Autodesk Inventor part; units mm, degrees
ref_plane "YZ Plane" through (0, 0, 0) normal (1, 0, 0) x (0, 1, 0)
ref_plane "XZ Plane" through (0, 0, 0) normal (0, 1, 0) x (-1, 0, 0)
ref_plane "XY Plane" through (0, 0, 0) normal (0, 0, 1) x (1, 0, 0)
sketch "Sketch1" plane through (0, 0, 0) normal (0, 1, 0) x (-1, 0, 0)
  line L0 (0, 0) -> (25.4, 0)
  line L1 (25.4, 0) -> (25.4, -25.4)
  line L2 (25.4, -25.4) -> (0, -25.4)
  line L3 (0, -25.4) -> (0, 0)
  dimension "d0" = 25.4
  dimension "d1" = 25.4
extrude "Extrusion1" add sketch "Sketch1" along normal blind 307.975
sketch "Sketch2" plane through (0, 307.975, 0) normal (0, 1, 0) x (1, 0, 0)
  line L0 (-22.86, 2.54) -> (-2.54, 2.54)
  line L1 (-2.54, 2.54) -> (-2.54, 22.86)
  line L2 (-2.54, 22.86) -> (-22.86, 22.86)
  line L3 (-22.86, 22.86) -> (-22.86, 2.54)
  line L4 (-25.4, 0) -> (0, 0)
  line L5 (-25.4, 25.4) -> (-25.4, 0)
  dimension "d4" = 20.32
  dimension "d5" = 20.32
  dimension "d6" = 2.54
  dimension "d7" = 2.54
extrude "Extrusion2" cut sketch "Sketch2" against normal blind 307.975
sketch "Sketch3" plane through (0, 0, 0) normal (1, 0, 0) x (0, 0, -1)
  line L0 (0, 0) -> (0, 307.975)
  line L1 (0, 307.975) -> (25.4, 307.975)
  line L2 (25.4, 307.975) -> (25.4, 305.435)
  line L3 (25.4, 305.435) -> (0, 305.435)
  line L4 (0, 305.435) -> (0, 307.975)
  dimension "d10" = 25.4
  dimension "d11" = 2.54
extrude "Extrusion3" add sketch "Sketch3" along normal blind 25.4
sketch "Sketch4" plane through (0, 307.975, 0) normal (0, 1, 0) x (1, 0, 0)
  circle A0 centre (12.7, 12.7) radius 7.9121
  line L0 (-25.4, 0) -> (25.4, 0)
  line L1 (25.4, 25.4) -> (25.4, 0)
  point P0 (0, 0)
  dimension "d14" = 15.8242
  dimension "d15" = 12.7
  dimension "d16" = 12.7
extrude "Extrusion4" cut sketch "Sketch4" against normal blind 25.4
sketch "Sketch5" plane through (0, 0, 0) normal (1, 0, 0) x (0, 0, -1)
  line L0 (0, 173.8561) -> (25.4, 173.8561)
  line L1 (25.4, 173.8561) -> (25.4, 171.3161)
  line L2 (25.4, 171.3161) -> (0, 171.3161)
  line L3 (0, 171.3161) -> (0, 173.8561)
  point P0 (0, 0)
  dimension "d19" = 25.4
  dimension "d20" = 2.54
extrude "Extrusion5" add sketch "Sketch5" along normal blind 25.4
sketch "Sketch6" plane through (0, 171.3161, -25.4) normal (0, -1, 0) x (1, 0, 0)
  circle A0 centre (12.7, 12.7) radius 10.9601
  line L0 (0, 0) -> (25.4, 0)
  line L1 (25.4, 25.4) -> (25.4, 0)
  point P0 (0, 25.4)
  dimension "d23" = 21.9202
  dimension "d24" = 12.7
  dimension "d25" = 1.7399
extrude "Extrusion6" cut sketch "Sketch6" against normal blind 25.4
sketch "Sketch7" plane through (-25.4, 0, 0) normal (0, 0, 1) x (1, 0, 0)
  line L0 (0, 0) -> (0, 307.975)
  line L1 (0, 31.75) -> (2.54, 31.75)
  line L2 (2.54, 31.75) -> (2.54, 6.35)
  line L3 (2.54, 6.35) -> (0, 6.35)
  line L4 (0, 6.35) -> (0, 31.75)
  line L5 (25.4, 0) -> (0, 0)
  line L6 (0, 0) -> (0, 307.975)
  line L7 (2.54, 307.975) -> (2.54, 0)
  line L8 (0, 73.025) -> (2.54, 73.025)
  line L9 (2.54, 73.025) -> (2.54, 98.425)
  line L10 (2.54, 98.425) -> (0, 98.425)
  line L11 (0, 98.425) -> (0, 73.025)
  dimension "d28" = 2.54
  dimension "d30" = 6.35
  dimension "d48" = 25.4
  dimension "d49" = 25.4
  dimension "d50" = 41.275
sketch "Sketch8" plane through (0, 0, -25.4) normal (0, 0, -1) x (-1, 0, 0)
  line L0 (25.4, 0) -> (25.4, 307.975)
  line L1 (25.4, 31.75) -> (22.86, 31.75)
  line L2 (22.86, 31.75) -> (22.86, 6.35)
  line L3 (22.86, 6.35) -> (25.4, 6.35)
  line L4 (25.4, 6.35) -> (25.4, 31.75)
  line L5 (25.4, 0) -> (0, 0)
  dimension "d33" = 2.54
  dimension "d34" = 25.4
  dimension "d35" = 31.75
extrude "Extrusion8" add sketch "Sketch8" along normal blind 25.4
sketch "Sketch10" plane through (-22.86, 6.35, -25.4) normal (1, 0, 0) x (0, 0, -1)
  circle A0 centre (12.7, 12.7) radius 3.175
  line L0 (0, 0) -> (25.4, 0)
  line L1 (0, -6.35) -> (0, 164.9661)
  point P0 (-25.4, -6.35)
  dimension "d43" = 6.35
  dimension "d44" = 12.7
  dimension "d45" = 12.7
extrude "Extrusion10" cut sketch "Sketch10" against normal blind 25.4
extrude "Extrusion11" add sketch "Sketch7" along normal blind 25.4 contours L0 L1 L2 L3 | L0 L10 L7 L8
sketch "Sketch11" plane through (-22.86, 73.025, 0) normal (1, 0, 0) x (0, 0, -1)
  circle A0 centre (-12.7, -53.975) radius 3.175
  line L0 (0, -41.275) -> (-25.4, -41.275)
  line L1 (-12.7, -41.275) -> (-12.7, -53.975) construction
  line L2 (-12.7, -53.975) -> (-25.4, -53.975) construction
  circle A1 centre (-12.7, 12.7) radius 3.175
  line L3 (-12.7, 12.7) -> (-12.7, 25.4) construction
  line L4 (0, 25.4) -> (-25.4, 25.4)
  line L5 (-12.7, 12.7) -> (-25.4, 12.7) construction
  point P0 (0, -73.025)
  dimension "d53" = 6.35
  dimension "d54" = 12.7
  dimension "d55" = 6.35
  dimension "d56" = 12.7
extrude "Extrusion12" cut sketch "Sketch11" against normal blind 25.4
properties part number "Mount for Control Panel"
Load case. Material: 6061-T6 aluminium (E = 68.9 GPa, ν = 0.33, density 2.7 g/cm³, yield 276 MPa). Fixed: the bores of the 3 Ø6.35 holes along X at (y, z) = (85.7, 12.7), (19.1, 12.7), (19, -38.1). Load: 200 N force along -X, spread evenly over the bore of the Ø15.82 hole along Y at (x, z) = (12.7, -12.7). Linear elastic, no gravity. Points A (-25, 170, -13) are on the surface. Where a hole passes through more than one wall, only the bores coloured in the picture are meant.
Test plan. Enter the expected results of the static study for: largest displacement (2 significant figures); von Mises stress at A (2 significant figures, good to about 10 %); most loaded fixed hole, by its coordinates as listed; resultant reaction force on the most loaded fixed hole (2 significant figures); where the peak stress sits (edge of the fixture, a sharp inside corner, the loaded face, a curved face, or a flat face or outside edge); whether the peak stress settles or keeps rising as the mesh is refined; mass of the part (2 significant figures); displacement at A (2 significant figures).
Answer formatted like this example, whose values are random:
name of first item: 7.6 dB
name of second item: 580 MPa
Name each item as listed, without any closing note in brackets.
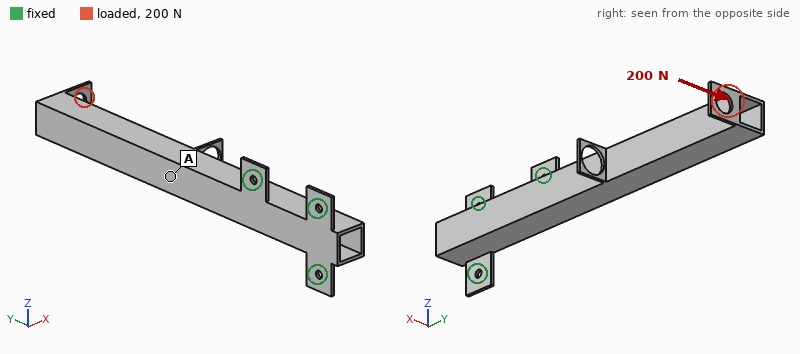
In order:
largest displacement: 1.5 mm
von Mises stress at A: 17 MPa
most loaded fixed hole, by its coordinates as listed: (85.7, 12.7)
resultant reaction force on the most loaded fixed hole: 840 N
where the peak stress sits: edge of the fixture
whether the peak stress settles or keeps rising as the mesh is refined: keeps rising
mass of the part: 210 g
displacement at A: 0.55 mm
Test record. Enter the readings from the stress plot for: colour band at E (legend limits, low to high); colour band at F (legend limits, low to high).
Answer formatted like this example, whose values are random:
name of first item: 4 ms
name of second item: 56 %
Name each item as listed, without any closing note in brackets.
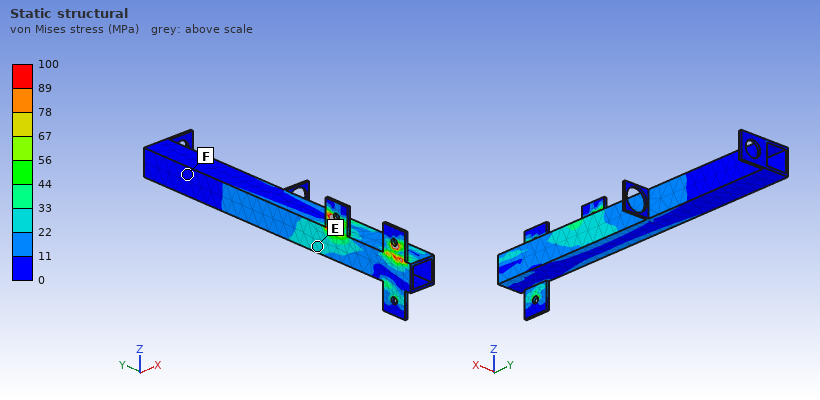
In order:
colour band at E: 22 to 33 MPa
colour band at F: 0 to 11 MPa
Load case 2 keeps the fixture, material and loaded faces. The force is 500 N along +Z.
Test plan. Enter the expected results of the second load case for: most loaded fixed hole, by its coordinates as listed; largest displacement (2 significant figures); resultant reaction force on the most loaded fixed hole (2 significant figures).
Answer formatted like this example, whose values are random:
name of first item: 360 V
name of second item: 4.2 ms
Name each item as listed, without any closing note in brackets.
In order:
most loaded fixed hole, by its coordinates as listed: (85.7, 12.7)
largest displacement: 2.3 mm
resultant reaction force on the most loaded fixed hole: 2.0 kN
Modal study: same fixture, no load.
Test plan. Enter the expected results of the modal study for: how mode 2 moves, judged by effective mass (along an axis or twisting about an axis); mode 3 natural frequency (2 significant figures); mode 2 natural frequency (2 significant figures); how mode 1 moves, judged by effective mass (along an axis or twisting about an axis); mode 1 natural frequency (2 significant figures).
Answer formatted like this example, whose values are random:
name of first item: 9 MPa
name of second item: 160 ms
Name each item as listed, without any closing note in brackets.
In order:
how mode 2 moves, judged by effective mass: along Z
mode 3 natural frequency: 1300 Hz
mode 2 natural frequency: 410 Hz
how mode 1 moves, judged by effective mass: along X
mode 1 natural frequency: 260 Hz
